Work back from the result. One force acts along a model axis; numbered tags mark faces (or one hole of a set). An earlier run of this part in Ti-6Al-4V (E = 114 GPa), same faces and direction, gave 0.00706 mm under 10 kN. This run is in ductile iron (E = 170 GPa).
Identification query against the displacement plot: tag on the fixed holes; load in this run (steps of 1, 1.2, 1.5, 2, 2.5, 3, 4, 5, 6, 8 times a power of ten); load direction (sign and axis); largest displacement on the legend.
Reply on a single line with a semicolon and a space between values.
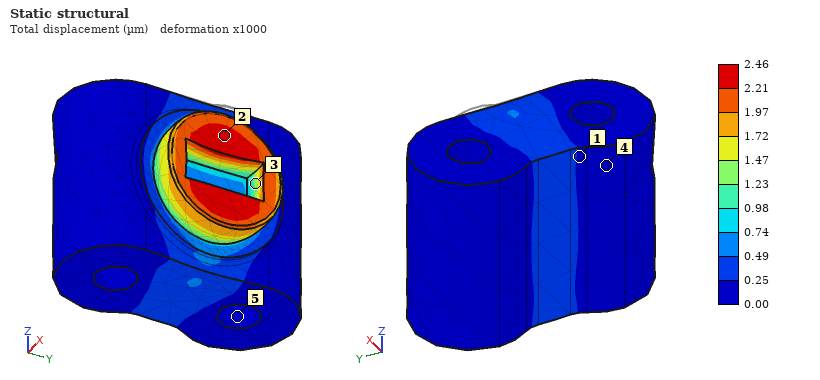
5; 5 kN; -X; 2.46 µm
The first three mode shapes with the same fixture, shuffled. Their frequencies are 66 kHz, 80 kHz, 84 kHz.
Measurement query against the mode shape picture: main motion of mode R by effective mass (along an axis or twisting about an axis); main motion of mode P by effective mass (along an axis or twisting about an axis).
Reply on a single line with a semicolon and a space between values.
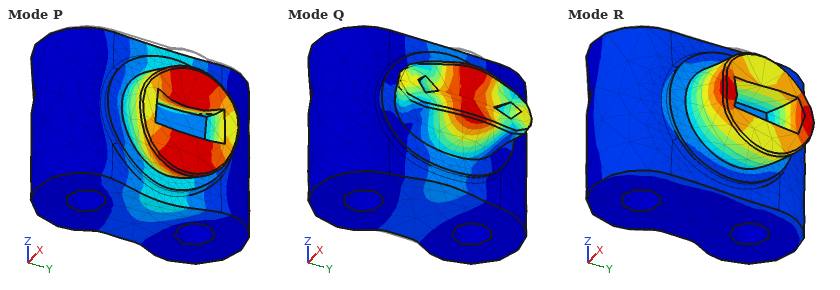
along Y; along Z
